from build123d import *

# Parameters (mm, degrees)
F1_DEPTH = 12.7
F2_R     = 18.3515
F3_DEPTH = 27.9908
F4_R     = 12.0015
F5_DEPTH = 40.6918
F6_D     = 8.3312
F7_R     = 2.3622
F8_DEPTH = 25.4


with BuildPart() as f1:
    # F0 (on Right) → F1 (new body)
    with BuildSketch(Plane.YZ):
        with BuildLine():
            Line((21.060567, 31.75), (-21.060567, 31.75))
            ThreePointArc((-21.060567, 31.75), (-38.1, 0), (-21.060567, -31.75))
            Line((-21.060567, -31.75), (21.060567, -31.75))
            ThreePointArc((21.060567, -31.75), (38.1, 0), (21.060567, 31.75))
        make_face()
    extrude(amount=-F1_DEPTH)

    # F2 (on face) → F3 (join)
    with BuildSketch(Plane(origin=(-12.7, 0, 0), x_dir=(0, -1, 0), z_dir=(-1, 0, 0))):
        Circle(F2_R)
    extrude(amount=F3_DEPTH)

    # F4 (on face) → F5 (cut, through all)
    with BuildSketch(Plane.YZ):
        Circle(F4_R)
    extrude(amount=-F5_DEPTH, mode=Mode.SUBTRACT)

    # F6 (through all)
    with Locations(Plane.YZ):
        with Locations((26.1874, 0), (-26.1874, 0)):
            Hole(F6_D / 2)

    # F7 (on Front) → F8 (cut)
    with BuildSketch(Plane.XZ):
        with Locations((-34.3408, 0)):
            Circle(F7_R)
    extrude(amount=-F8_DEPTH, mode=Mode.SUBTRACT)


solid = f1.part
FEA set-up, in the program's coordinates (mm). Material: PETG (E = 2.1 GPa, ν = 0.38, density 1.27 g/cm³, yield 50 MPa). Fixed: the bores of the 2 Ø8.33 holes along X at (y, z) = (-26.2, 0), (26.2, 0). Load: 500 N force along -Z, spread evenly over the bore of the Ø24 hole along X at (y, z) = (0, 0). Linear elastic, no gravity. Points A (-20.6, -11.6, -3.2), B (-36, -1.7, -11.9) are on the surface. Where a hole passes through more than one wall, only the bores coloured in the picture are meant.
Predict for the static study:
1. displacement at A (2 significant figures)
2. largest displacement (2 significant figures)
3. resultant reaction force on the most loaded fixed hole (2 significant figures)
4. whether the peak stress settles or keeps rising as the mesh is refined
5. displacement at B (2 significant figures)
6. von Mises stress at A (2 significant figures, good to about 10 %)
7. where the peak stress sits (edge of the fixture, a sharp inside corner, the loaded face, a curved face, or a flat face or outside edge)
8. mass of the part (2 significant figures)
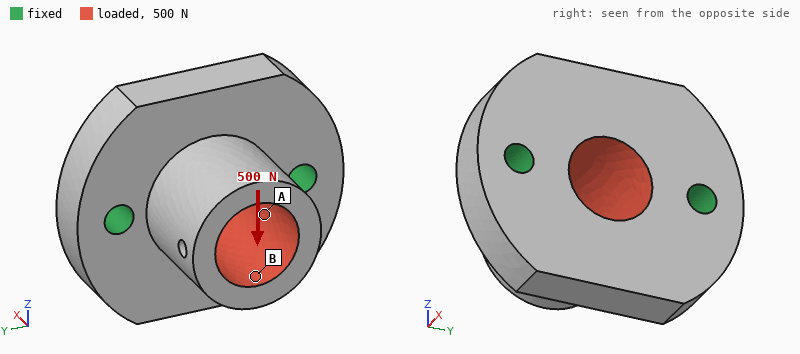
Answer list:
0.050 mm
0.13 mm
250 N
keeps rising
0.11 mm
1.7 MPa
edge of the fixture
80 g
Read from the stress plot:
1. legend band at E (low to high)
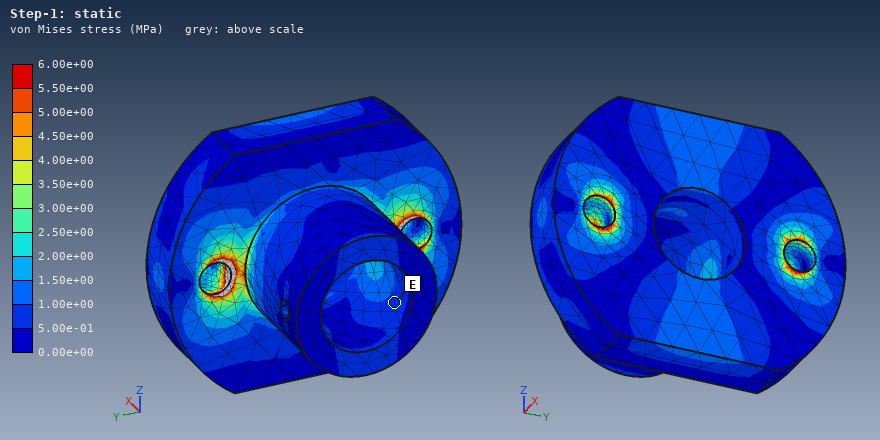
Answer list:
5.00e-01 to 1.00e+00 MPa
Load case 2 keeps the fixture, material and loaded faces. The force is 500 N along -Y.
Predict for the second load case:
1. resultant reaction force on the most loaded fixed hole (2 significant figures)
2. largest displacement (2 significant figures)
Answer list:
290 N
47 µm
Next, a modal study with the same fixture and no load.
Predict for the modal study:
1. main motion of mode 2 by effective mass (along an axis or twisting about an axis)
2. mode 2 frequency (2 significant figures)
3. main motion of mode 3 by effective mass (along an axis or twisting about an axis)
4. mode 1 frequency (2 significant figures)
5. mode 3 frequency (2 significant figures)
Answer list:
along X
2600 Hz
along Y
1600 Hz
3300 Hz
